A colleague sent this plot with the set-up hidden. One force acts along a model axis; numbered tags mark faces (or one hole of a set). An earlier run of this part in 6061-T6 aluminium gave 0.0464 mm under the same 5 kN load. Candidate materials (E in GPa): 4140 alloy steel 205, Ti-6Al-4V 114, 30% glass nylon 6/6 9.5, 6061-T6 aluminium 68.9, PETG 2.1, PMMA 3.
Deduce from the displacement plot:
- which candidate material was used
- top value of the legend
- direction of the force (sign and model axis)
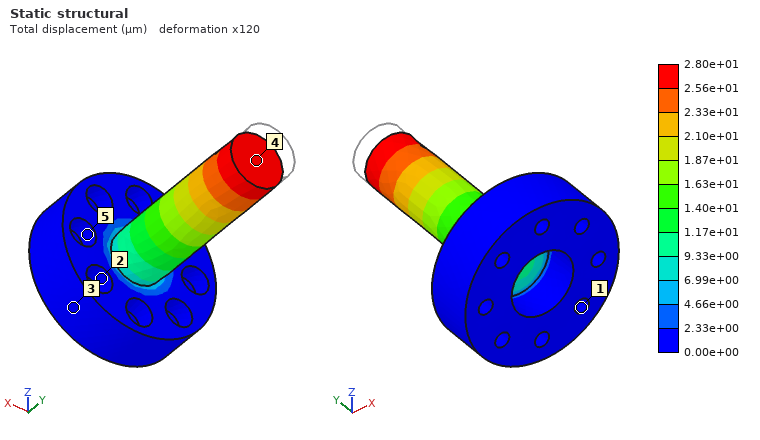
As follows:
Ti-6Al-4V
2.80e+01 µm
-Y
